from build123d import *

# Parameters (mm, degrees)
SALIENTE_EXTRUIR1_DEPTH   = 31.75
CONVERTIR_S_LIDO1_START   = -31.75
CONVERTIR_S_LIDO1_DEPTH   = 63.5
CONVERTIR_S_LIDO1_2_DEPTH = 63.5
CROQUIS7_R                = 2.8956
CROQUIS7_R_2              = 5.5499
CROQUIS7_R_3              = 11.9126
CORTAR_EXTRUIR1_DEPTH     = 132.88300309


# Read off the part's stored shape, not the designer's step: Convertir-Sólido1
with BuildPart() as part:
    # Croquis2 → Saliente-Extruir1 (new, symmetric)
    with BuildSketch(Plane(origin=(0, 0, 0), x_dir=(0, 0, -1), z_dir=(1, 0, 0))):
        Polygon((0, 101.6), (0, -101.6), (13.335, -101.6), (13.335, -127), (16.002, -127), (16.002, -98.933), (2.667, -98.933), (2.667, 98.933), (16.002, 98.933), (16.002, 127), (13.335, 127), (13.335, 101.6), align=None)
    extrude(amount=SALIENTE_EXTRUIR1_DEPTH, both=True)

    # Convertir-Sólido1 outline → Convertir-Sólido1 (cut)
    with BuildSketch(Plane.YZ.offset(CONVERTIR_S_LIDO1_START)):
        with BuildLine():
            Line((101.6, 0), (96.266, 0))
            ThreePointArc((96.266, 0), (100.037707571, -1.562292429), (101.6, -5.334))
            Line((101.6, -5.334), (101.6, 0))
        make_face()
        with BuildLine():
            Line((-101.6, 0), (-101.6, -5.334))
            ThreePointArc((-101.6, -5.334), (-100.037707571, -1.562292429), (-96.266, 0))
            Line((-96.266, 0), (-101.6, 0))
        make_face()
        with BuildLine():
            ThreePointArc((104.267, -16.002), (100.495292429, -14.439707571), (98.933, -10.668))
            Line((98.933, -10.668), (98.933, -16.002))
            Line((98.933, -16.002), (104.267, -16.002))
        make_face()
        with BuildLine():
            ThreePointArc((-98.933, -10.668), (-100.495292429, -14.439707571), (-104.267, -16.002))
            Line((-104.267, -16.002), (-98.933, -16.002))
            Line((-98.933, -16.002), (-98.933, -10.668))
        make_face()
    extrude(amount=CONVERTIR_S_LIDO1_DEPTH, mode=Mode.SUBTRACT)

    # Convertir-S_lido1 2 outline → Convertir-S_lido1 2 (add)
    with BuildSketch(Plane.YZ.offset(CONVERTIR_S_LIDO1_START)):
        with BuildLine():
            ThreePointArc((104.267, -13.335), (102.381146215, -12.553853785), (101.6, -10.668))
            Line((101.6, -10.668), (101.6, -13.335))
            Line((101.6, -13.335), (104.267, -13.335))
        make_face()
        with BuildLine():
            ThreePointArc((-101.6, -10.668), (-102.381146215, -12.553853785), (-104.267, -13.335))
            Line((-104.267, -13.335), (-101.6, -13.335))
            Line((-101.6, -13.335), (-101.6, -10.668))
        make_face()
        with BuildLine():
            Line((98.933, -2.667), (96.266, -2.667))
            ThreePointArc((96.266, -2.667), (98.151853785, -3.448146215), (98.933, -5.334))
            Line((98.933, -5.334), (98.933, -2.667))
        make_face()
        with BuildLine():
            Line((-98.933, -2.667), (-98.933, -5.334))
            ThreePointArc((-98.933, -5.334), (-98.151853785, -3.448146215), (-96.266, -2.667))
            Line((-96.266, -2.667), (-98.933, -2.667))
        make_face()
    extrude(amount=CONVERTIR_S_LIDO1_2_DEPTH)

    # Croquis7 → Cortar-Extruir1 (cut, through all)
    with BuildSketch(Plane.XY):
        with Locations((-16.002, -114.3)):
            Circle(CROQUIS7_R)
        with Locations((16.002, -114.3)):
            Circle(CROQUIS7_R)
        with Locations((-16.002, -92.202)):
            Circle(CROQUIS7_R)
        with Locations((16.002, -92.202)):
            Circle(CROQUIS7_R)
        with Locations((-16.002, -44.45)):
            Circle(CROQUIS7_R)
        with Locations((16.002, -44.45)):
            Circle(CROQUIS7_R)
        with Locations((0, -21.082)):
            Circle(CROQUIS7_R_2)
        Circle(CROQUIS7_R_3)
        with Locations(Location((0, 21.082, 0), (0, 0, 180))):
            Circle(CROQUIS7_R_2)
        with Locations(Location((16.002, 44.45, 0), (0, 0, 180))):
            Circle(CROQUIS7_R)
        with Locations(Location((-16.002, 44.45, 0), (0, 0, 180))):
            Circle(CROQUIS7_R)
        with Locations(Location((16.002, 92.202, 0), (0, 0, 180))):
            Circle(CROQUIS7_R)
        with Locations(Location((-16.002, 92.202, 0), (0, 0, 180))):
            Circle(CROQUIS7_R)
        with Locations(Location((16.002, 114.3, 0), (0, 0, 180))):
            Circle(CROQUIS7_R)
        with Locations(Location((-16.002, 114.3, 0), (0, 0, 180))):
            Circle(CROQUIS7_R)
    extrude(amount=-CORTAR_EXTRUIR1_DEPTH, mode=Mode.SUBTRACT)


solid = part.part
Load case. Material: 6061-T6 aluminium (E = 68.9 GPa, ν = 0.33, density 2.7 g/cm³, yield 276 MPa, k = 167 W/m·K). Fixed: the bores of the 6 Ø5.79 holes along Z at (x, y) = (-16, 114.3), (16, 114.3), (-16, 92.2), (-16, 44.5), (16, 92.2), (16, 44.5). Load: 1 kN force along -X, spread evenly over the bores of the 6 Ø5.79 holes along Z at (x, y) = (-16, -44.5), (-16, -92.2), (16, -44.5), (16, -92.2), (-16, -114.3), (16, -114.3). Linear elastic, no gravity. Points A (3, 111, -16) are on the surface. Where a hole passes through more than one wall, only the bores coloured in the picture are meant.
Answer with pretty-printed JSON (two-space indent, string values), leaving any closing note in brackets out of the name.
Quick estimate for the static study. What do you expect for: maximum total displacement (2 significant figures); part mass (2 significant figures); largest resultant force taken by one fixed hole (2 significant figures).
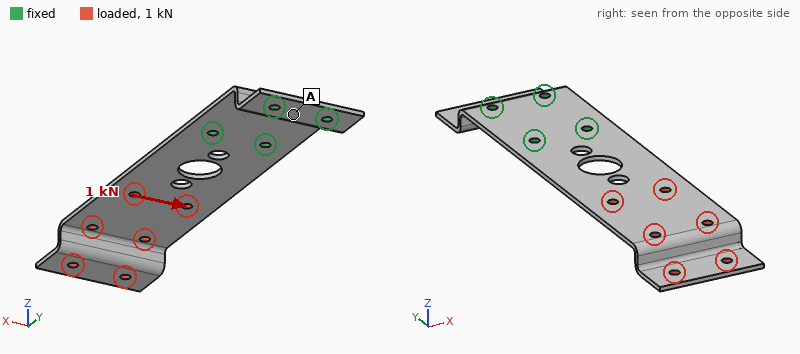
{
  "maximum total displacement": "2.2 mm",
  "part mass": "120 g",
  "largest resultant force taken by one fixed hole": "2.7 kN"
}
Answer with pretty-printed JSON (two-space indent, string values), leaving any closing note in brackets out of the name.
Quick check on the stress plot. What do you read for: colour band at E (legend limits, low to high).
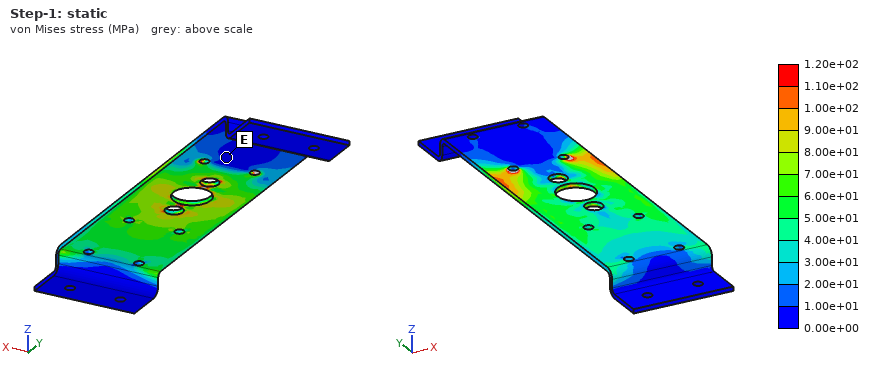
{
  "colour band at E": "0.00e+00 to 1.00e+01 MPa"
}
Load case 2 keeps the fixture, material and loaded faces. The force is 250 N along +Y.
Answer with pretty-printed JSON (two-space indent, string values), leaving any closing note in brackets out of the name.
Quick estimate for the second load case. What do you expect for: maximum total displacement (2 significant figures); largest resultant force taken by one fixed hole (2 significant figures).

{
  "maximum total displacement": "2.7 mm",
  "largest resultant force taken by one fixed hole": "110 N"
}
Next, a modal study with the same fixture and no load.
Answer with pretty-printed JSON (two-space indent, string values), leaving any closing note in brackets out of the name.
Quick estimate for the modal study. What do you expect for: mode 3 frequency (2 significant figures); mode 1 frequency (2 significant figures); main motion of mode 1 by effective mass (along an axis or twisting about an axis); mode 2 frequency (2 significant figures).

{
  "mode 3 frequency": "450 Hz",
  "mode 1 frequency": "65 Hz",
  "main motion of mode 1 by effective mass": "along Z",
  "mode 2 frequency": "340 Hz"
}
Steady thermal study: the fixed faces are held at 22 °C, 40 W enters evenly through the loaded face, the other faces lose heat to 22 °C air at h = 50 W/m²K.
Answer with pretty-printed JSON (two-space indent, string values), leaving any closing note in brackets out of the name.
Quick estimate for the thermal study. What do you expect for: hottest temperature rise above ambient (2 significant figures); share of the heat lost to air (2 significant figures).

{
  "hottest temperature rise above ambient": "52 K",
  "share of the heat lost to air": "85 %"
}
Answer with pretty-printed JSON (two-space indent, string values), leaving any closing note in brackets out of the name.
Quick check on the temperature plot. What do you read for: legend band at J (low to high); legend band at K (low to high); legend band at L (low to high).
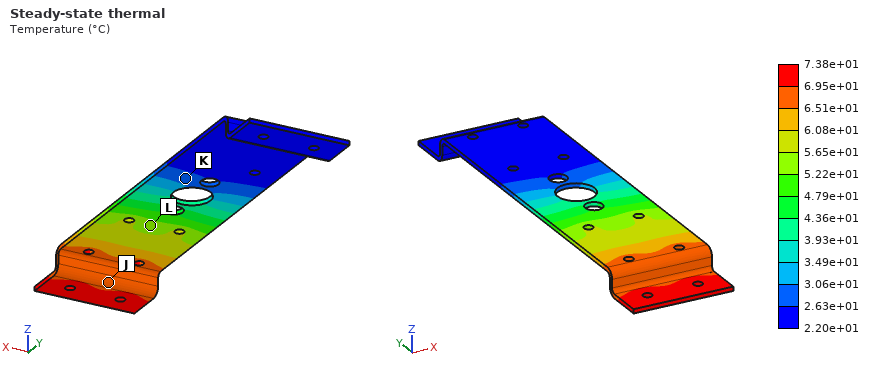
{
  "legend band at J": "6.51e+01 to 6.95e+01 °C",
  "legend band at K": "2.63e+01 to 3.06e+01 °C",
  "legend band at L": "5.22e+01 to 5.65e+01 °C"
}
